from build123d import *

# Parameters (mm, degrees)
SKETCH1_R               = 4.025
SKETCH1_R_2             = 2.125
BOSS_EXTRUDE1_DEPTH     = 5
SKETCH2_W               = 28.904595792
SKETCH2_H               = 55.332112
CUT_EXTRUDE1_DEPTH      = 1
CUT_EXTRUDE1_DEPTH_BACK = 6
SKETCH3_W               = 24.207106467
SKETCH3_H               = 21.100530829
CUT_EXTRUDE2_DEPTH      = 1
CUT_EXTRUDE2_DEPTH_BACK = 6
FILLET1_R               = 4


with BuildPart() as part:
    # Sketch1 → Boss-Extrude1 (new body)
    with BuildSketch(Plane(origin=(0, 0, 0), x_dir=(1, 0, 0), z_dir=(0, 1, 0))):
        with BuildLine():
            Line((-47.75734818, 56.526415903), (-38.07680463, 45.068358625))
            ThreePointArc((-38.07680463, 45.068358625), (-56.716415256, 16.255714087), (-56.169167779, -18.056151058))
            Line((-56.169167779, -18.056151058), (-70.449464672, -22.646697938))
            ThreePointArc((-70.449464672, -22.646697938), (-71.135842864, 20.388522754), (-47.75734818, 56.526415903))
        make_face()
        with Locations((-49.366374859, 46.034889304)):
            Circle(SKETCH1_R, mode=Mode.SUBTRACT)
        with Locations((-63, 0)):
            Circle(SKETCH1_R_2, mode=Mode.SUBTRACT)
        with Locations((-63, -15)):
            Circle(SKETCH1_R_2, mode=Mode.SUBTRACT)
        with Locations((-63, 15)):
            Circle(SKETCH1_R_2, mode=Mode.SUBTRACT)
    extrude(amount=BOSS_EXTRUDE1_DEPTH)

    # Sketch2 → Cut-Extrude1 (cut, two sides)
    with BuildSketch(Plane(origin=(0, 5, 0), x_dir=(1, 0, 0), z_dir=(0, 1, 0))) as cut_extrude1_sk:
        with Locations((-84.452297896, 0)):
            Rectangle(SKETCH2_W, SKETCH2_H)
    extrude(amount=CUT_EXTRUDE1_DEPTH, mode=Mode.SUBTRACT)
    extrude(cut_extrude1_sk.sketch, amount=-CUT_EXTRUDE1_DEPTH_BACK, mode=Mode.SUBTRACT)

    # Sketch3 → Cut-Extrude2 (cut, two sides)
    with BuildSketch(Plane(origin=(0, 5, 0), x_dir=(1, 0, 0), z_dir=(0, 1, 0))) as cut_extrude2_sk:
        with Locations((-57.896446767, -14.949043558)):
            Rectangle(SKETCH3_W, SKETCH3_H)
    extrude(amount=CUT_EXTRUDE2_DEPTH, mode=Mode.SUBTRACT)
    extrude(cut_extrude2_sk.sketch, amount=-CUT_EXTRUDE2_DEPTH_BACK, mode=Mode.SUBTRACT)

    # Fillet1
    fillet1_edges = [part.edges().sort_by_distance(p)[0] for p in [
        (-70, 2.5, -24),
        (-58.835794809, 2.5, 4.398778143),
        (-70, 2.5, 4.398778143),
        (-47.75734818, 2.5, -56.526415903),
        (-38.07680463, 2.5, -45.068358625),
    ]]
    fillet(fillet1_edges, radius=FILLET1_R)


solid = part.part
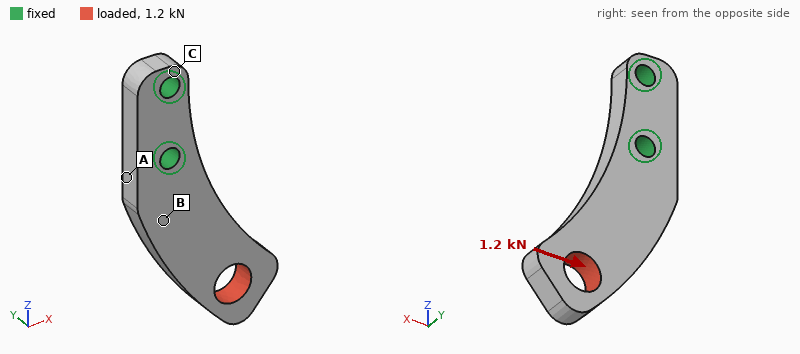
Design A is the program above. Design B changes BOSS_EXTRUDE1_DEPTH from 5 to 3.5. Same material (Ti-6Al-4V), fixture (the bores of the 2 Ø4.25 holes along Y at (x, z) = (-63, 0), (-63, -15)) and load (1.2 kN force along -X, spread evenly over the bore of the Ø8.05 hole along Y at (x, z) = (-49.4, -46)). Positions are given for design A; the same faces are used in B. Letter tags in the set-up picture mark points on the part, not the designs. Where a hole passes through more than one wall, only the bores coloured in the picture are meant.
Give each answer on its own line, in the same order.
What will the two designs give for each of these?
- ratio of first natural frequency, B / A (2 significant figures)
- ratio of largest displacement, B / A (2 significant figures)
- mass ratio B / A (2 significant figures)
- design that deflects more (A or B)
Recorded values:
0.72
1.4
0.70
B
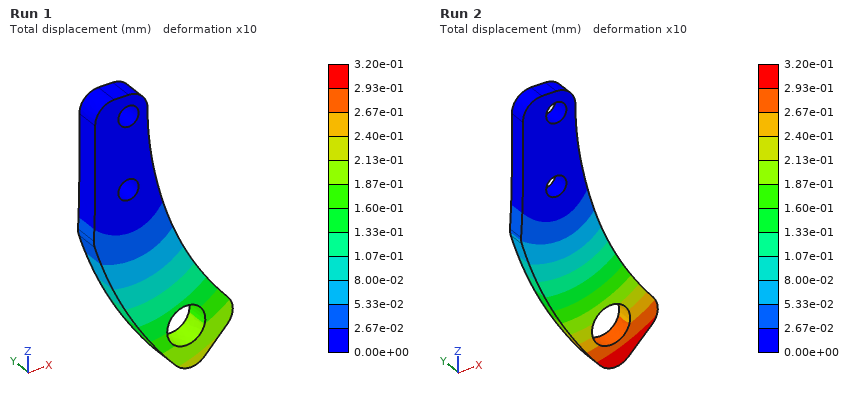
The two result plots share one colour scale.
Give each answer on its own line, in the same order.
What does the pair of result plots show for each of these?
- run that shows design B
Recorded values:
Run 2
